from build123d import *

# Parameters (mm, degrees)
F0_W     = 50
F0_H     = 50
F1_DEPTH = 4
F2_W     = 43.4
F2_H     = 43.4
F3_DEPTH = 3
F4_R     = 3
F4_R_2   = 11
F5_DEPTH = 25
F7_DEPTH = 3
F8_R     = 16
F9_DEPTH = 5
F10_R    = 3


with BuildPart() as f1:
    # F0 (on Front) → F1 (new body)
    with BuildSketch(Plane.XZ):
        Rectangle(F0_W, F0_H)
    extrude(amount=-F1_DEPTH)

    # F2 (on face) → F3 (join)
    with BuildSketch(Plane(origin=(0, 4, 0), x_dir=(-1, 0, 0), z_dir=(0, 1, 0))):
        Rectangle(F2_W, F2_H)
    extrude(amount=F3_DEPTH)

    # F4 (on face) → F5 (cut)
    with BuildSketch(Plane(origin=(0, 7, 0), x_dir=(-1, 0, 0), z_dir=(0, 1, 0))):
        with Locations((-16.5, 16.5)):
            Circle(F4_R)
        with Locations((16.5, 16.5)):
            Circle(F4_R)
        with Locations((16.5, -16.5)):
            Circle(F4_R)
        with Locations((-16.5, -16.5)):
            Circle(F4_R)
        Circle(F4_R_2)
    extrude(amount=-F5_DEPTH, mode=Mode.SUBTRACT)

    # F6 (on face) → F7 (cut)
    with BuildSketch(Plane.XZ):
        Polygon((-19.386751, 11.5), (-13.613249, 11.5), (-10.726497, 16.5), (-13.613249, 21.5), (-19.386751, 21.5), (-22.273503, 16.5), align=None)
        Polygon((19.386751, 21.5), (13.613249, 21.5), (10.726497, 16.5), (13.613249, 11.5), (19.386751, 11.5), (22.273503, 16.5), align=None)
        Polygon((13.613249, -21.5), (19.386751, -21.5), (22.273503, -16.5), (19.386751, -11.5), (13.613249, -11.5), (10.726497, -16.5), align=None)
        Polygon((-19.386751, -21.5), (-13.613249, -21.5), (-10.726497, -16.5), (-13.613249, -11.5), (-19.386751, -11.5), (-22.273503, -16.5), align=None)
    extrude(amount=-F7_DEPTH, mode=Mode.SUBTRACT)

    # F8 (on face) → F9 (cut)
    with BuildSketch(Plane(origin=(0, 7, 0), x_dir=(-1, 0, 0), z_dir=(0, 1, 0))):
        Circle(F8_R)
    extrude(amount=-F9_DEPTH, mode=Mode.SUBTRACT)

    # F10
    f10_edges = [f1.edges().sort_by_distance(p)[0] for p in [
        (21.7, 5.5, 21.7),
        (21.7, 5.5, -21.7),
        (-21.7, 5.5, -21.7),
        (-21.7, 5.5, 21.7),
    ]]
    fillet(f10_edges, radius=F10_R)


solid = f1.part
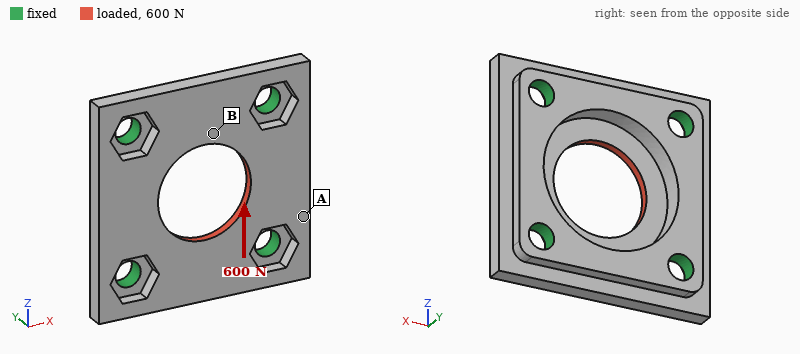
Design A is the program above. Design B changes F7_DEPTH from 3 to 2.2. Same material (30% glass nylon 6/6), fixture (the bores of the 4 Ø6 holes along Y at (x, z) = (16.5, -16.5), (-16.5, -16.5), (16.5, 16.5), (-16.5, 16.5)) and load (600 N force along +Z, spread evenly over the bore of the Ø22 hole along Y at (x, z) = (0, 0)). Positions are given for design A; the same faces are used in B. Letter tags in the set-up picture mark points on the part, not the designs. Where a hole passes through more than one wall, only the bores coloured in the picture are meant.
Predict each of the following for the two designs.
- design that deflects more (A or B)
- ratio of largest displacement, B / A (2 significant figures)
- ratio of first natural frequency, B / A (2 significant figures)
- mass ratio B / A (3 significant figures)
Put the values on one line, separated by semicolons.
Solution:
A; 0.89; 1.1; 1.02
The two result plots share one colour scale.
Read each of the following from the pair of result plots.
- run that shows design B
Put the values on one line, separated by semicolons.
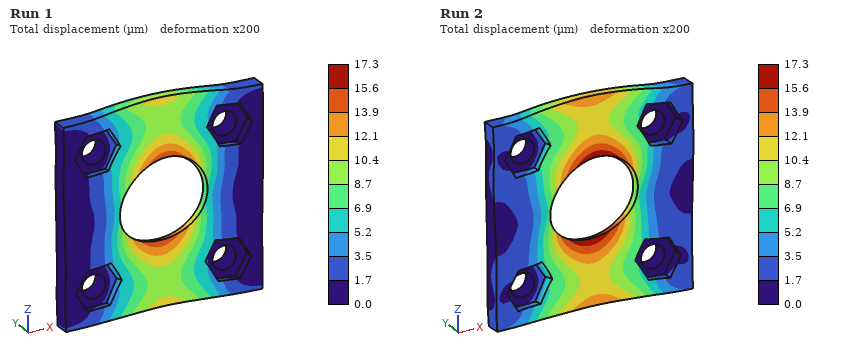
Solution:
Run 1
